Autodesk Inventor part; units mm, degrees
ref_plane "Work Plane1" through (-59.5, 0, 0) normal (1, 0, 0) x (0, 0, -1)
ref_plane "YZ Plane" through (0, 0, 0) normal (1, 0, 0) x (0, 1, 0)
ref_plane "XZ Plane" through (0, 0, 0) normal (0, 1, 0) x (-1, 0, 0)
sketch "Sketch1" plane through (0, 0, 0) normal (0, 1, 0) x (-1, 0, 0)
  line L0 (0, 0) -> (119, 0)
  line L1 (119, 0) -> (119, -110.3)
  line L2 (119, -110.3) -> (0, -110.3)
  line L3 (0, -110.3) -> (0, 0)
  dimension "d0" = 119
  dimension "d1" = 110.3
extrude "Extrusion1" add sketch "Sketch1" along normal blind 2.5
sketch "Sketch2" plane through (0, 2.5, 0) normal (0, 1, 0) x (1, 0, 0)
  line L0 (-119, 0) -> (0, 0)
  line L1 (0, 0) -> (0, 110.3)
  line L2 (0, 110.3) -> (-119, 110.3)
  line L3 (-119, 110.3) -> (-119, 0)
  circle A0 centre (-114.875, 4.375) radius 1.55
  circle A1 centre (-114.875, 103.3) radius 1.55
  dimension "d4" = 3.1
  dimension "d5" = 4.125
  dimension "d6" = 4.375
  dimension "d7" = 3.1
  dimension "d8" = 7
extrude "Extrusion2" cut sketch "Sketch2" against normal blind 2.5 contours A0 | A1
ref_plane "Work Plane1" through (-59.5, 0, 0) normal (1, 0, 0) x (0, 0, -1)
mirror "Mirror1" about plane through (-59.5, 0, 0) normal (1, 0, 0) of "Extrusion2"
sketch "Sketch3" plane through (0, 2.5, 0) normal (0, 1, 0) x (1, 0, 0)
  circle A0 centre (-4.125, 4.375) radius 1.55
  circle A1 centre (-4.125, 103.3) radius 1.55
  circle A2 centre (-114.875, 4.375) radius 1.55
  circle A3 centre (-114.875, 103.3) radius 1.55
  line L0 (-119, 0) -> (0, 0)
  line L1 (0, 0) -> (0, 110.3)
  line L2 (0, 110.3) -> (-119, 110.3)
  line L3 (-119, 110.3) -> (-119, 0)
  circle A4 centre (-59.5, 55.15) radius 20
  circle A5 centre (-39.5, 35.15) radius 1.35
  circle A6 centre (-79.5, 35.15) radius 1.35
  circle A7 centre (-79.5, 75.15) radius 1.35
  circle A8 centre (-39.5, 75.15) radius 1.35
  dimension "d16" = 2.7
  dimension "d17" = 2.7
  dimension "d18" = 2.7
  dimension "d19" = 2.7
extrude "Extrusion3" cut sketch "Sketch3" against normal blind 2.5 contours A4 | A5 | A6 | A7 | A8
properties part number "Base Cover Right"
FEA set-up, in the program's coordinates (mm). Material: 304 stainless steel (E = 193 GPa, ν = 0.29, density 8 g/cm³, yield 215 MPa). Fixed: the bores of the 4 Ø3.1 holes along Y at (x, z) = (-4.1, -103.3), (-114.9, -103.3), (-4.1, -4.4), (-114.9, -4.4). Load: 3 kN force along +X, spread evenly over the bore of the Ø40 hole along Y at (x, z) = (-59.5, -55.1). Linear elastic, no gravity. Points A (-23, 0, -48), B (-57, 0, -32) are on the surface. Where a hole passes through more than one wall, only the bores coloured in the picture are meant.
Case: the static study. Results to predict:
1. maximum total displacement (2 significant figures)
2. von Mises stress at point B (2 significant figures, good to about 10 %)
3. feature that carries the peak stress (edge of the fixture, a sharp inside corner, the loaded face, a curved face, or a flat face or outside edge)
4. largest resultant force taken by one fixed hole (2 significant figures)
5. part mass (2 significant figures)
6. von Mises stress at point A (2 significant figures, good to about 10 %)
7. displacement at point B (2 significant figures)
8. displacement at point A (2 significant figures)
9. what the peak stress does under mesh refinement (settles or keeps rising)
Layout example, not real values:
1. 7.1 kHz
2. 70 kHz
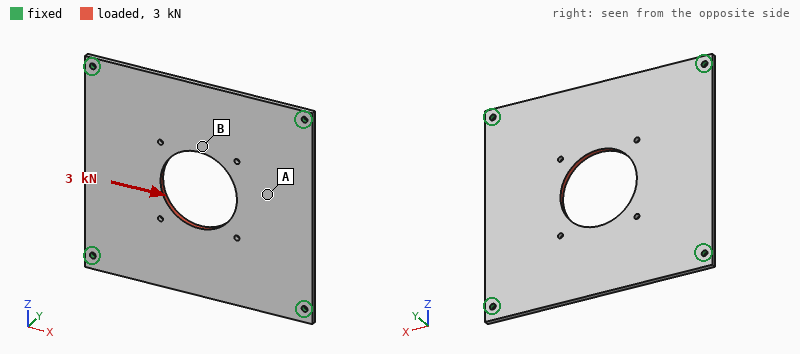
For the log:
1. 5.7 µm
2. 15 MPa
3. edge of the fixture
4. 850 N
5. 240 g
6. 5.1 MPa
7. 4.5 µm
8. 5.0 µm
9. keeps rising
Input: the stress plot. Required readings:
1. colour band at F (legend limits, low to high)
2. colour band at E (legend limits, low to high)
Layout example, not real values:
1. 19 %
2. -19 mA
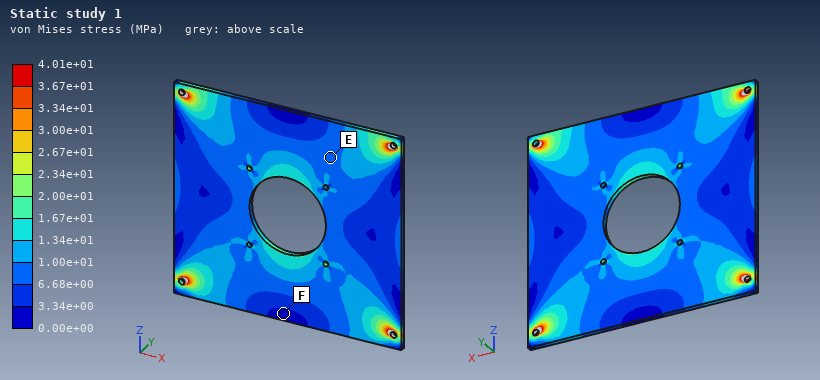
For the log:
1. 0.00e+00 to 3.34e+00 MPa
2. 6.68e+00 to 1.00e+01 MPa
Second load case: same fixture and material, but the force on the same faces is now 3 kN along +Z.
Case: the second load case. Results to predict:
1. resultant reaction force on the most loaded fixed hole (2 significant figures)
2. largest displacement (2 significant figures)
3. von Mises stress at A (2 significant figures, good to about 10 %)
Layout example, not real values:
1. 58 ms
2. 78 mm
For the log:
1. 860 N
2. 6.8 µm
3. 12 MPa
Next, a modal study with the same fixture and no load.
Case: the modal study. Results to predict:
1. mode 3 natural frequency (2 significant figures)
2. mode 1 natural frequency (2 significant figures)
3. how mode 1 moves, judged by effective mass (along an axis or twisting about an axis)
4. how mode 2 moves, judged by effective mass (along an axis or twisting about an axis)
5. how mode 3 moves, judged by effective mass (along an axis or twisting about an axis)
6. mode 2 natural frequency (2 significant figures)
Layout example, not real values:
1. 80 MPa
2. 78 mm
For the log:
1. 1300 Hz
2. 680 Hz
3. along Y
4. twisting about X
5. twisting about Z
6. 1100 Hz
